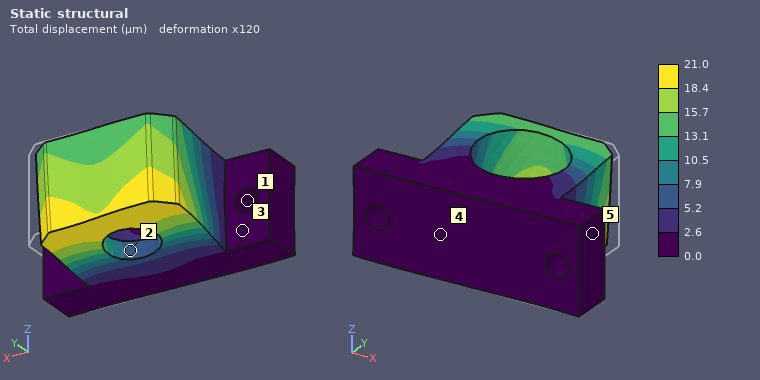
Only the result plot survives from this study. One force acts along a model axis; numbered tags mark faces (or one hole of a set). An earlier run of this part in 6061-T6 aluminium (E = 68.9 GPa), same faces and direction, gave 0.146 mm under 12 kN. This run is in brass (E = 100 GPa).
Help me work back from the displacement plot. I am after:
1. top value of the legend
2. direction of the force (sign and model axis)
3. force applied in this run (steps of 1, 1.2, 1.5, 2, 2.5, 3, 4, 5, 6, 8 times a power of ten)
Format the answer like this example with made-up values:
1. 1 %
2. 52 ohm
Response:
1. 21.0 µm
2. -X
3. 2.5 kN
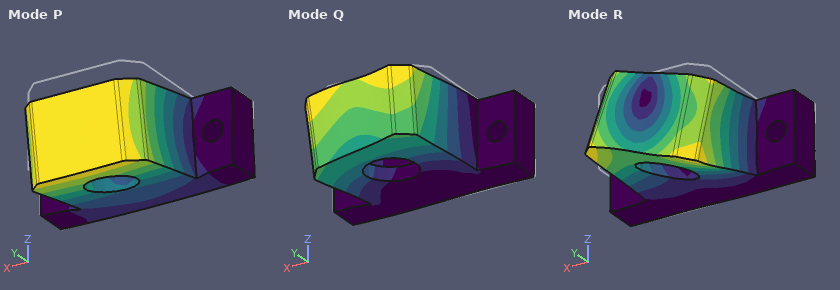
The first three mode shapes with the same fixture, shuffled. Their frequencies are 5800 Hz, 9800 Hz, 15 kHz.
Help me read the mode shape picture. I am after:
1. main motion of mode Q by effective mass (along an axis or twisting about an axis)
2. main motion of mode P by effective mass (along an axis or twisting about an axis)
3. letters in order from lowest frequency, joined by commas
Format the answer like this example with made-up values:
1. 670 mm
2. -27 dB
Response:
1. along X
2. along Z
3. P, Q, R
